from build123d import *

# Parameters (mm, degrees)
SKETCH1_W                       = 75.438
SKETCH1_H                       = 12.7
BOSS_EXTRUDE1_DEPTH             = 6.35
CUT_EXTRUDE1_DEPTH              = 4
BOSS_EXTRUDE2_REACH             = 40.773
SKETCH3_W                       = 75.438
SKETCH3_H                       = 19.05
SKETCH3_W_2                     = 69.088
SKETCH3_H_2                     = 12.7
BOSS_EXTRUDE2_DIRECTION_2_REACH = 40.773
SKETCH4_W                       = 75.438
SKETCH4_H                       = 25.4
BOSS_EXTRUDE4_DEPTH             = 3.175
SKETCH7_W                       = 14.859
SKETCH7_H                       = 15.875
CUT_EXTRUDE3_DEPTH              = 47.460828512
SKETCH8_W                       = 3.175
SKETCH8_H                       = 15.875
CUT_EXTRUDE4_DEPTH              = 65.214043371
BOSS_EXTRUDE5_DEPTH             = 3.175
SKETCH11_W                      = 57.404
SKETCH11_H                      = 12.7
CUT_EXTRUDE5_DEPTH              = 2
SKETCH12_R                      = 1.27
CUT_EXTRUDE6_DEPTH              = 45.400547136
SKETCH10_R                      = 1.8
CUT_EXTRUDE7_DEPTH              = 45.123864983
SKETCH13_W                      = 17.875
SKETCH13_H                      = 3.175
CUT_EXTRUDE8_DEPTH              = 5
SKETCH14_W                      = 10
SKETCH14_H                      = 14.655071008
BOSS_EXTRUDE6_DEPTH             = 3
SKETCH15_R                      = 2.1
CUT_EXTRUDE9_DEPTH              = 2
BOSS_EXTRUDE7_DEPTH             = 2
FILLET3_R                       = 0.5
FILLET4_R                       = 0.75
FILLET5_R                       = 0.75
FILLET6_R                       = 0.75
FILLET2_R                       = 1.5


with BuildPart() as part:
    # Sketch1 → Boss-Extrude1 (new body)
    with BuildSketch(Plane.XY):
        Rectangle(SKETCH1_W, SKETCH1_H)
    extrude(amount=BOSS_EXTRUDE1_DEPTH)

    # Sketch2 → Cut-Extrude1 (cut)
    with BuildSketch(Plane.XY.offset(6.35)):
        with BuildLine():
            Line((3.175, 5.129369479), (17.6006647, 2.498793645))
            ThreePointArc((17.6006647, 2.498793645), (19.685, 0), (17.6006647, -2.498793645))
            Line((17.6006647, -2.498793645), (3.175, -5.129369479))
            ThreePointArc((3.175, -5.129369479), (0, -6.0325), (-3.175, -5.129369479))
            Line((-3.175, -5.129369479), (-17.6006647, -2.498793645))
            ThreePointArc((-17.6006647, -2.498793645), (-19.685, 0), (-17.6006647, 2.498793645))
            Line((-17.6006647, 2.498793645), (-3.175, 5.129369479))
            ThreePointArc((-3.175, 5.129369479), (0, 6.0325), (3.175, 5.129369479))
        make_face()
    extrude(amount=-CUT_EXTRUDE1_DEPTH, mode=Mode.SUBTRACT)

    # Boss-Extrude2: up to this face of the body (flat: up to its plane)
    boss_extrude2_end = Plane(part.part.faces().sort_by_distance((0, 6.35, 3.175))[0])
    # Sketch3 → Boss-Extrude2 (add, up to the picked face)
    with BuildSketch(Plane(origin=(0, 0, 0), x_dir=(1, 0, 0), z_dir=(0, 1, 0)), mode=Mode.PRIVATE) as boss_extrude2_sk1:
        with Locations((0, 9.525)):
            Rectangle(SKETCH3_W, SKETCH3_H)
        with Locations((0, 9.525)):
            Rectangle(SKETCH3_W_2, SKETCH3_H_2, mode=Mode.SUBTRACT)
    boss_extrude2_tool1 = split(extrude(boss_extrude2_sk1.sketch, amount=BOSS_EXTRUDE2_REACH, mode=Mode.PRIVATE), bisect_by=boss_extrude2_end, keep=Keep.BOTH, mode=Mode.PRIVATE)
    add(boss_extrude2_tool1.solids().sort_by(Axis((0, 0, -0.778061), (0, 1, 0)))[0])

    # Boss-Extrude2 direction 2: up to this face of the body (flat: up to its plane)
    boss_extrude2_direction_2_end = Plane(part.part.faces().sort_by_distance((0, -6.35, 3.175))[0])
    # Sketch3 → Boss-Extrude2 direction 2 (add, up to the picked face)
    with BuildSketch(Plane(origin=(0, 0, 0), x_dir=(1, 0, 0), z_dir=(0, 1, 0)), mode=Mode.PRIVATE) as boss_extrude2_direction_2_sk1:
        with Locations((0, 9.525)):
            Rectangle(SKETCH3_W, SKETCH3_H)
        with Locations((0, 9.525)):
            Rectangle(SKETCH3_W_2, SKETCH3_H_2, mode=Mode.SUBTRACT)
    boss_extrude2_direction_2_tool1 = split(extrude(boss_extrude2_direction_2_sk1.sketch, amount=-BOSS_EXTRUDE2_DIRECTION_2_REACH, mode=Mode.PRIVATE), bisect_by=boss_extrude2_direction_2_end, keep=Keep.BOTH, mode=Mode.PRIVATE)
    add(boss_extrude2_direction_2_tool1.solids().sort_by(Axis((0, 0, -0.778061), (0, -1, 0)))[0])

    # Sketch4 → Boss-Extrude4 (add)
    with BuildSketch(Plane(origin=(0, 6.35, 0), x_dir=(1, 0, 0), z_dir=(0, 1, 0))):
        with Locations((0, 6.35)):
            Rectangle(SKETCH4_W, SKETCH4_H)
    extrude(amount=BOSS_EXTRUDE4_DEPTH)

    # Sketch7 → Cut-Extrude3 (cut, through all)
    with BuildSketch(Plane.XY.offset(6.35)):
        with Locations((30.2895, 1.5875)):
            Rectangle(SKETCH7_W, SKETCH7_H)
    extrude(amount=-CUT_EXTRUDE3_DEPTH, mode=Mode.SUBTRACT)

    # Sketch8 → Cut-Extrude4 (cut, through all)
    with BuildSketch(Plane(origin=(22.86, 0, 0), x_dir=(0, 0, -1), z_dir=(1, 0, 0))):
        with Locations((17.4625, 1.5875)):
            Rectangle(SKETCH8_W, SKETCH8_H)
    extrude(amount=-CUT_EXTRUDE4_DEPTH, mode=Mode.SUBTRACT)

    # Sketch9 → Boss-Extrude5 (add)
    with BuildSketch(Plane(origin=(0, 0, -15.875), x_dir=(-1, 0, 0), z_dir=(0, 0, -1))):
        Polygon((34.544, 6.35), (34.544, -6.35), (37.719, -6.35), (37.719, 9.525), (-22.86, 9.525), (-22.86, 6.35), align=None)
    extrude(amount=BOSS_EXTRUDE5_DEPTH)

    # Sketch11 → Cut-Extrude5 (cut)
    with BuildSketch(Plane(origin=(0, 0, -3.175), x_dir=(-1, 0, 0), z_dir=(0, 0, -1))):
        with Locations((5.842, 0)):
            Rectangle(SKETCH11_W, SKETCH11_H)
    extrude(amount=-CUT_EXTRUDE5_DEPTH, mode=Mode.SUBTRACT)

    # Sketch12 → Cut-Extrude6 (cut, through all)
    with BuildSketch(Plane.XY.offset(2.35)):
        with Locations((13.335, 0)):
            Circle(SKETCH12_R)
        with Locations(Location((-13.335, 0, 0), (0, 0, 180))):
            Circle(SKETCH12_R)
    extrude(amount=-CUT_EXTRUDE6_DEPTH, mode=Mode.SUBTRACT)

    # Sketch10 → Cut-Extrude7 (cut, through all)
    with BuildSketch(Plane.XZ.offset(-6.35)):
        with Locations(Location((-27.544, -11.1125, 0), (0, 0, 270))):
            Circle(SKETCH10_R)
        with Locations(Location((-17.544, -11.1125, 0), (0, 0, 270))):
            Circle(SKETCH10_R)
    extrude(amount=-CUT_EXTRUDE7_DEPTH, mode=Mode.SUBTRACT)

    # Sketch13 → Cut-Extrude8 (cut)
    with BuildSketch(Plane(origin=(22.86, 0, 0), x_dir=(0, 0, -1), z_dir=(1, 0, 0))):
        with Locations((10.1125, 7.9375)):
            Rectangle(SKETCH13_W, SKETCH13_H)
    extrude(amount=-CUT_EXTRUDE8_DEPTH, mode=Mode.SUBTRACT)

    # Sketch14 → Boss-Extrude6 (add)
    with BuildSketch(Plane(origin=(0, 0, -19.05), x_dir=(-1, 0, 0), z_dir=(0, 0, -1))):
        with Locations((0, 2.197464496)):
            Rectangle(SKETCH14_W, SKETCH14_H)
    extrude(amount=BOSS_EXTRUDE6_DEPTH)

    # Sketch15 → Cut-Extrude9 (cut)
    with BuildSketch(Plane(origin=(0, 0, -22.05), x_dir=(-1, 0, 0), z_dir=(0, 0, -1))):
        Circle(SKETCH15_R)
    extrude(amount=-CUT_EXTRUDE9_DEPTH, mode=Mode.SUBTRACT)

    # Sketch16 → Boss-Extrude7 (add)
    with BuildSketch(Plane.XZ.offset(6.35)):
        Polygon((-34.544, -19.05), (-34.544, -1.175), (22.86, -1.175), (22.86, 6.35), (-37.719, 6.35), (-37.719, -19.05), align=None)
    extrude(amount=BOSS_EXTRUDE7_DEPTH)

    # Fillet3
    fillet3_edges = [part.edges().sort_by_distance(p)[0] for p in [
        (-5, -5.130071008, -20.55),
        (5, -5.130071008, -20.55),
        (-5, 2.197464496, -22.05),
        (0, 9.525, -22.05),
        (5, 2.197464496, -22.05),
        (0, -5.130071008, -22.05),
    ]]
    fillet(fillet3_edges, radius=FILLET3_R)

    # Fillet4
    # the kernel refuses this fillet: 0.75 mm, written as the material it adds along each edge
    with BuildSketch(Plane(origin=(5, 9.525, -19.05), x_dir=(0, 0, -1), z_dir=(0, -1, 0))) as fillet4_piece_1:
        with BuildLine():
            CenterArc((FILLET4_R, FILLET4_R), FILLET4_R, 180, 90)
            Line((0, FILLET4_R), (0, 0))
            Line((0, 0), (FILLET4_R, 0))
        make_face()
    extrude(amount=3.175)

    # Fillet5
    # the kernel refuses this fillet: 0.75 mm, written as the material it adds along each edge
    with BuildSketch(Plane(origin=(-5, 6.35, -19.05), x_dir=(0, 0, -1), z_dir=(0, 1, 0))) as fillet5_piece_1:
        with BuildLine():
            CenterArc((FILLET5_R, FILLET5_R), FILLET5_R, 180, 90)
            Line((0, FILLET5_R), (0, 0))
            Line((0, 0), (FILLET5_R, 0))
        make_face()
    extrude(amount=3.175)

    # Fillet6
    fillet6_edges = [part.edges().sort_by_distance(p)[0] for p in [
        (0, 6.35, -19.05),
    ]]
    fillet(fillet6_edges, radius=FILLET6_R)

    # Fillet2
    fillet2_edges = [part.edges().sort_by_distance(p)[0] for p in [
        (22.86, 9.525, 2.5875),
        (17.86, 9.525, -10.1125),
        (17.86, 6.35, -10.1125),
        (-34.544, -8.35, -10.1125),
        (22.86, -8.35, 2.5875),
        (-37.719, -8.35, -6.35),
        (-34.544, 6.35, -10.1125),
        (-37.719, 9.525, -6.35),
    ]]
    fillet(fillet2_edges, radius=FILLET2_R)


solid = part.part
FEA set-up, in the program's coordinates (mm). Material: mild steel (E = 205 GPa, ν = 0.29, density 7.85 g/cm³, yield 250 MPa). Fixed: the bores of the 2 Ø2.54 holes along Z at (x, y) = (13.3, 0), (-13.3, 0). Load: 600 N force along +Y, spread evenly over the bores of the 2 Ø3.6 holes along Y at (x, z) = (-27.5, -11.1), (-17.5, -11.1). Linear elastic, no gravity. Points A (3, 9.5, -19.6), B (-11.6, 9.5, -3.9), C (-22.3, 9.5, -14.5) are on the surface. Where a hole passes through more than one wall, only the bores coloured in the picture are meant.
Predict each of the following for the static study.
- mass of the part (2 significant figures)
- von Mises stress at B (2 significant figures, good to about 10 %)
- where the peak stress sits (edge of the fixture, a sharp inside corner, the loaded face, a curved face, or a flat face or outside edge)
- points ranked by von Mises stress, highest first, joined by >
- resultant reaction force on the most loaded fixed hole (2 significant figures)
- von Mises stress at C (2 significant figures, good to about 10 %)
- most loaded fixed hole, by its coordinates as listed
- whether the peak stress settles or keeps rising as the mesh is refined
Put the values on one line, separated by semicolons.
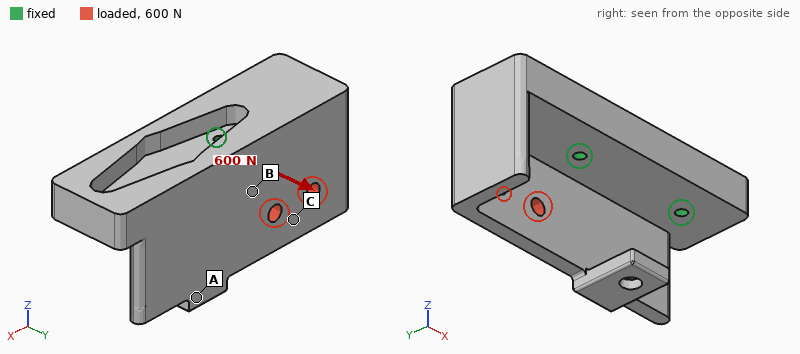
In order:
88 g; 43 MPa; edge of the fixture; B > C > A; 780 N; 25 MPa; (-13.3, 0); keeps rising
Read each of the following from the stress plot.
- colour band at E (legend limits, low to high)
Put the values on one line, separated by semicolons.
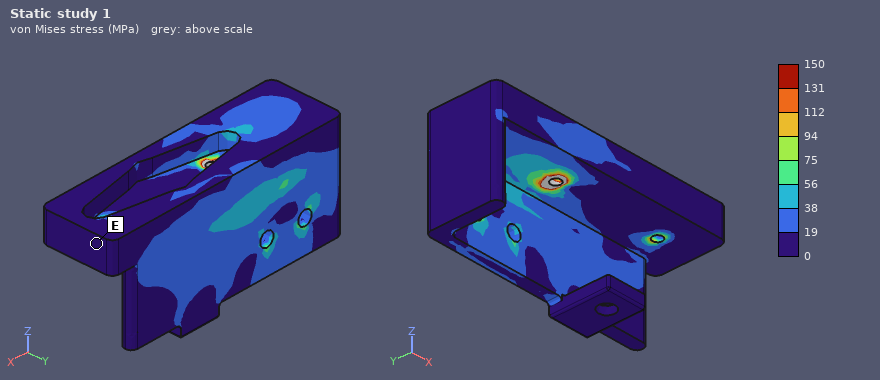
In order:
0 to 19 MPa
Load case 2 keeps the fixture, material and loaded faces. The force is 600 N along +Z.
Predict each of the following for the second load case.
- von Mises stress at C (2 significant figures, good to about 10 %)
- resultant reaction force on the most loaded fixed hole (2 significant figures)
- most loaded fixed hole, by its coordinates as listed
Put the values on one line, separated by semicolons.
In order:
9.4 MPa; 760 N; (-13.3, 0)
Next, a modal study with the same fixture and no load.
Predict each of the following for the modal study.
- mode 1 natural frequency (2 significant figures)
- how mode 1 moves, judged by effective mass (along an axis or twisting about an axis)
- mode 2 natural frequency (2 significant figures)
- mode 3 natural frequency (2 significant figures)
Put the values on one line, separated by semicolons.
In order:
3600 Hz; along Y; 5100 Hz; 6400 Hz
